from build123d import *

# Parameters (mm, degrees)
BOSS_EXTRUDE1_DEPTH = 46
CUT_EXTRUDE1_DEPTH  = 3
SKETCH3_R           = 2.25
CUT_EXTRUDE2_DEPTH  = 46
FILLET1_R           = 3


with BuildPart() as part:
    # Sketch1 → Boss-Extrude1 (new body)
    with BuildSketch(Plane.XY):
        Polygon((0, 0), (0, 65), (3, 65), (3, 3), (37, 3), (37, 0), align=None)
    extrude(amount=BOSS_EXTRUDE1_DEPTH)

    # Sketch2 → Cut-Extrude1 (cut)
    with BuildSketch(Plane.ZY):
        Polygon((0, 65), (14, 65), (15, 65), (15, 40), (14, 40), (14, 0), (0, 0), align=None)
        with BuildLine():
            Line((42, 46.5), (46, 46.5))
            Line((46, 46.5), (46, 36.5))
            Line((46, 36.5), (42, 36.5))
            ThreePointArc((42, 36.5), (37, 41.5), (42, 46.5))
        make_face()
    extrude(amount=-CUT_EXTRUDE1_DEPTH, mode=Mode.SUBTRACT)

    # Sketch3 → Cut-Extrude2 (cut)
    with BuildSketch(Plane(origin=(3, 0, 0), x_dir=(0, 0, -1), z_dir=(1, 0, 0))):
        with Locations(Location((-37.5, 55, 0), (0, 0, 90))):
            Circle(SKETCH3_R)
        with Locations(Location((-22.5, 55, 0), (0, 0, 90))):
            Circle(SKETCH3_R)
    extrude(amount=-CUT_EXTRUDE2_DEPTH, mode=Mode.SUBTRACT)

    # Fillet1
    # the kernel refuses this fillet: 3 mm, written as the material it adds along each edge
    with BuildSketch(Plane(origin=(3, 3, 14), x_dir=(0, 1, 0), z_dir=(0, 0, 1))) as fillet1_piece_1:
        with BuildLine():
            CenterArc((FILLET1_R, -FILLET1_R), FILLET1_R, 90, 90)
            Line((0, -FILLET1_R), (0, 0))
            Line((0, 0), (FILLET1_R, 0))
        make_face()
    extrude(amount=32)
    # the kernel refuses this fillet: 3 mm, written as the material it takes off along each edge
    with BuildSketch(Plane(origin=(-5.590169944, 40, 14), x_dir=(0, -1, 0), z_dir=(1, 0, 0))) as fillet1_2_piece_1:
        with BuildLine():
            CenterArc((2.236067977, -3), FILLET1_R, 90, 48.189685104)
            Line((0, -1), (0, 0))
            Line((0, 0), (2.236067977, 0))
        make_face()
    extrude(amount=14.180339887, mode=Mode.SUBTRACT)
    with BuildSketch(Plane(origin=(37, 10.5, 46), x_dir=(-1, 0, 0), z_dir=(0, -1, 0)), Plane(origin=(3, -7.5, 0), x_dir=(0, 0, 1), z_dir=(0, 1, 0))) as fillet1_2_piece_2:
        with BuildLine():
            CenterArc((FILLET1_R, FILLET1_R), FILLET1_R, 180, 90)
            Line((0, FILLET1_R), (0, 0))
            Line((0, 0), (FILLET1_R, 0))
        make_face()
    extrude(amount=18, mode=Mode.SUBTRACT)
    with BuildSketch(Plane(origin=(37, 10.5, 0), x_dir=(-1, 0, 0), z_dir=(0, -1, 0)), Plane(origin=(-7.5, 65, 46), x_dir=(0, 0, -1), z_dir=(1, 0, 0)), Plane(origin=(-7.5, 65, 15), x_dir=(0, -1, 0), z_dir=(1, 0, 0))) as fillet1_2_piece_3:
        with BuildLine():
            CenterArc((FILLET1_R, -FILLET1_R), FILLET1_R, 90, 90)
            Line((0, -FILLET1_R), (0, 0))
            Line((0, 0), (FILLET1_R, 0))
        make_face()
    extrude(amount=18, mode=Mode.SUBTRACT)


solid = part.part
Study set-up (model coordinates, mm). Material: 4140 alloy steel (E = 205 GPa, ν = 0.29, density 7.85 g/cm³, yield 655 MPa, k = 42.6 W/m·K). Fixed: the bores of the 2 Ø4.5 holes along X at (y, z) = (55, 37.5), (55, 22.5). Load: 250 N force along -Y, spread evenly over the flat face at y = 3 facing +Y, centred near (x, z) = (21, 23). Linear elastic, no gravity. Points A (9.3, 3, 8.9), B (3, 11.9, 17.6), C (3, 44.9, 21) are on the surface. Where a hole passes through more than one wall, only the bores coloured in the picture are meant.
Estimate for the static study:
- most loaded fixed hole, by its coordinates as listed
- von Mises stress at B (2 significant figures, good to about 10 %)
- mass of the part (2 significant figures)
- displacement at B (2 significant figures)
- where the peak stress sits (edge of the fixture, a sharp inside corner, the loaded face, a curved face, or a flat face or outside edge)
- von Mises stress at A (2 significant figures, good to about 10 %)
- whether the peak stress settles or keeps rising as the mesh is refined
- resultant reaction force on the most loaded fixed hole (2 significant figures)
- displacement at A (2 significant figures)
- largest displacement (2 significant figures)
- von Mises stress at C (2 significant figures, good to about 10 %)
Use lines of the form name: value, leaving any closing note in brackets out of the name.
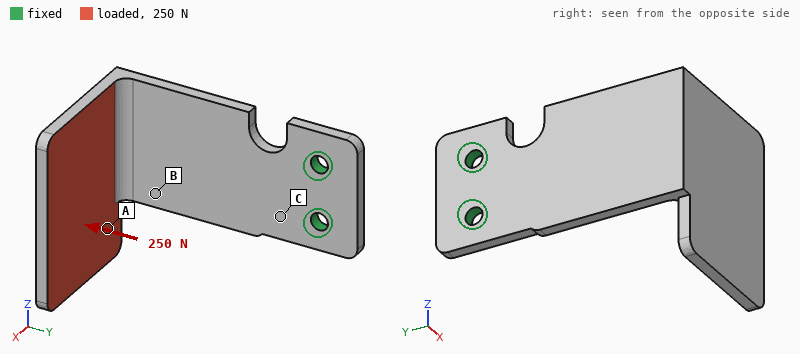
most loaded fixed hole, by its coordinates as listed: (55, 22.5)
von Mises stress at B: 110 MPa
mass of the part: 83 g
displacement at B: 0.35 mm
where the peak stress sits: edge of the fixture
von Mises stress at A: 22 MPa
whether the peak stress settles or keeps rising as the mesh is refined: keeps rising
resultant reaction force on the most loaded fixed hole: 230 N
displacement at A: 0.53 mm
largest displacement: 0.95 mm
von Mises stress at C: 130 MPa
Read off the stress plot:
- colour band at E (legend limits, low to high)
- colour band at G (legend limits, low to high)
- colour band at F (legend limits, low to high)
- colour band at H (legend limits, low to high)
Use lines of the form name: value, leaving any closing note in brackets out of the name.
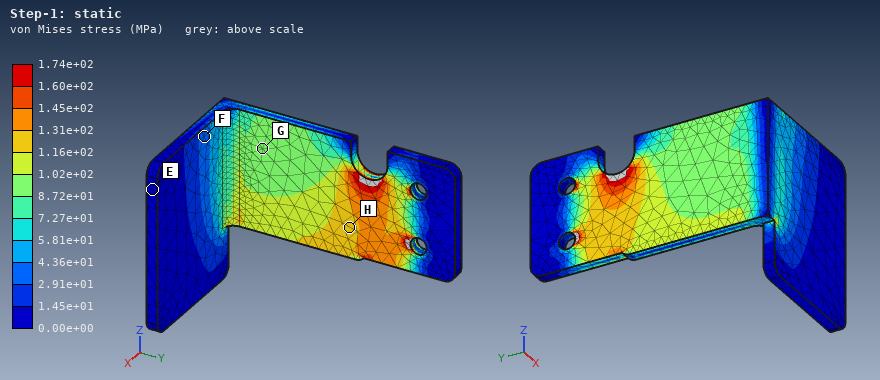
colour band at E: 0.00e+00 to 1.45e+01 MPa
colour band at G: 8.72e+01 to 1.02e+02 MPa
colour band at F: 2.91e+01 to 4.36e+01 MPa
colour band at H: 1.16e+02 to 1.31e+02 MPa
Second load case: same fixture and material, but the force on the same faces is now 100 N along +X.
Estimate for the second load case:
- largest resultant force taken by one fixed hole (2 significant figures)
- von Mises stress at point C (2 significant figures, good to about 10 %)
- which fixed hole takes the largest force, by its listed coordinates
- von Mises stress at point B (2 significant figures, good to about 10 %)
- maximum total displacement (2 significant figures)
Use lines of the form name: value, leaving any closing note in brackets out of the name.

largest resultant force taken by one fixed hole: 100 N
von Mises stress at point C: 110 MPa
which fixed hole takes the largest force, by its listed coordinates: (55, 22.5)
von Mises stress at point B: 24 MPa
maximum total displacement: 0.57 mm
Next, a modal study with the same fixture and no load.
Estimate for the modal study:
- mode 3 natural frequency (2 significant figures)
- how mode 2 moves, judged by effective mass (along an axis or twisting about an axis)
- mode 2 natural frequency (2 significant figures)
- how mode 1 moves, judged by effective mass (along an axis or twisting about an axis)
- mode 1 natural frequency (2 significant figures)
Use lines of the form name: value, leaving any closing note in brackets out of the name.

mode 3 natural frequency: 1200 Hz
how mode 2 moves, judged by effective mass: along Z
mode 2 natural frequency: 680 Hz
how mode 1 moves, judged by effective mass: along X
mode 1 natural frequency: 320 Hz
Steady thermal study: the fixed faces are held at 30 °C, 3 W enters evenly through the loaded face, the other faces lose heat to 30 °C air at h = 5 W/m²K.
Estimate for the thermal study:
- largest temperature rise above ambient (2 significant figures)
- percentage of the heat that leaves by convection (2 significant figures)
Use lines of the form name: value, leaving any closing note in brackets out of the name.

largest temperature rise above ambient: 45 K
percentage of the heat that leaves by convection: 25 %
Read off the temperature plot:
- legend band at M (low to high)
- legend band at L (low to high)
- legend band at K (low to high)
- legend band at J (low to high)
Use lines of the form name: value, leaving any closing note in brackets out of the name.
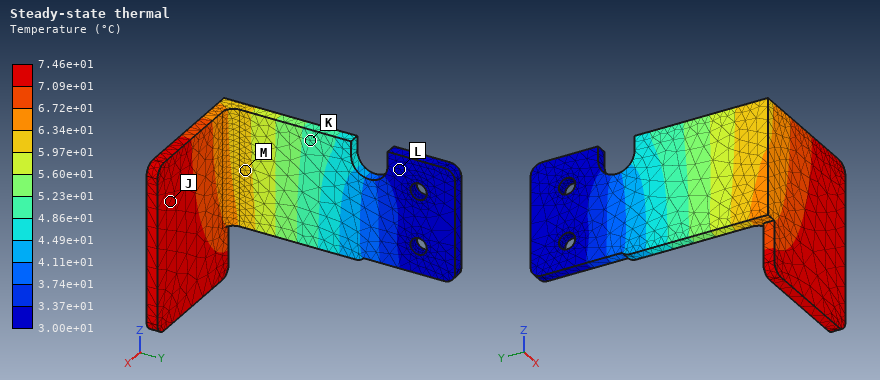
legend band at M: 5.97e+01 to 6.34e+01 °C
legend band at L: 3.00e+01 to 3.37e+01 °C
legend band at K: 4.86e+01 to 5.23e+01 °C
legend band at J: 7.09e+01 to 7.46e+01 °C
